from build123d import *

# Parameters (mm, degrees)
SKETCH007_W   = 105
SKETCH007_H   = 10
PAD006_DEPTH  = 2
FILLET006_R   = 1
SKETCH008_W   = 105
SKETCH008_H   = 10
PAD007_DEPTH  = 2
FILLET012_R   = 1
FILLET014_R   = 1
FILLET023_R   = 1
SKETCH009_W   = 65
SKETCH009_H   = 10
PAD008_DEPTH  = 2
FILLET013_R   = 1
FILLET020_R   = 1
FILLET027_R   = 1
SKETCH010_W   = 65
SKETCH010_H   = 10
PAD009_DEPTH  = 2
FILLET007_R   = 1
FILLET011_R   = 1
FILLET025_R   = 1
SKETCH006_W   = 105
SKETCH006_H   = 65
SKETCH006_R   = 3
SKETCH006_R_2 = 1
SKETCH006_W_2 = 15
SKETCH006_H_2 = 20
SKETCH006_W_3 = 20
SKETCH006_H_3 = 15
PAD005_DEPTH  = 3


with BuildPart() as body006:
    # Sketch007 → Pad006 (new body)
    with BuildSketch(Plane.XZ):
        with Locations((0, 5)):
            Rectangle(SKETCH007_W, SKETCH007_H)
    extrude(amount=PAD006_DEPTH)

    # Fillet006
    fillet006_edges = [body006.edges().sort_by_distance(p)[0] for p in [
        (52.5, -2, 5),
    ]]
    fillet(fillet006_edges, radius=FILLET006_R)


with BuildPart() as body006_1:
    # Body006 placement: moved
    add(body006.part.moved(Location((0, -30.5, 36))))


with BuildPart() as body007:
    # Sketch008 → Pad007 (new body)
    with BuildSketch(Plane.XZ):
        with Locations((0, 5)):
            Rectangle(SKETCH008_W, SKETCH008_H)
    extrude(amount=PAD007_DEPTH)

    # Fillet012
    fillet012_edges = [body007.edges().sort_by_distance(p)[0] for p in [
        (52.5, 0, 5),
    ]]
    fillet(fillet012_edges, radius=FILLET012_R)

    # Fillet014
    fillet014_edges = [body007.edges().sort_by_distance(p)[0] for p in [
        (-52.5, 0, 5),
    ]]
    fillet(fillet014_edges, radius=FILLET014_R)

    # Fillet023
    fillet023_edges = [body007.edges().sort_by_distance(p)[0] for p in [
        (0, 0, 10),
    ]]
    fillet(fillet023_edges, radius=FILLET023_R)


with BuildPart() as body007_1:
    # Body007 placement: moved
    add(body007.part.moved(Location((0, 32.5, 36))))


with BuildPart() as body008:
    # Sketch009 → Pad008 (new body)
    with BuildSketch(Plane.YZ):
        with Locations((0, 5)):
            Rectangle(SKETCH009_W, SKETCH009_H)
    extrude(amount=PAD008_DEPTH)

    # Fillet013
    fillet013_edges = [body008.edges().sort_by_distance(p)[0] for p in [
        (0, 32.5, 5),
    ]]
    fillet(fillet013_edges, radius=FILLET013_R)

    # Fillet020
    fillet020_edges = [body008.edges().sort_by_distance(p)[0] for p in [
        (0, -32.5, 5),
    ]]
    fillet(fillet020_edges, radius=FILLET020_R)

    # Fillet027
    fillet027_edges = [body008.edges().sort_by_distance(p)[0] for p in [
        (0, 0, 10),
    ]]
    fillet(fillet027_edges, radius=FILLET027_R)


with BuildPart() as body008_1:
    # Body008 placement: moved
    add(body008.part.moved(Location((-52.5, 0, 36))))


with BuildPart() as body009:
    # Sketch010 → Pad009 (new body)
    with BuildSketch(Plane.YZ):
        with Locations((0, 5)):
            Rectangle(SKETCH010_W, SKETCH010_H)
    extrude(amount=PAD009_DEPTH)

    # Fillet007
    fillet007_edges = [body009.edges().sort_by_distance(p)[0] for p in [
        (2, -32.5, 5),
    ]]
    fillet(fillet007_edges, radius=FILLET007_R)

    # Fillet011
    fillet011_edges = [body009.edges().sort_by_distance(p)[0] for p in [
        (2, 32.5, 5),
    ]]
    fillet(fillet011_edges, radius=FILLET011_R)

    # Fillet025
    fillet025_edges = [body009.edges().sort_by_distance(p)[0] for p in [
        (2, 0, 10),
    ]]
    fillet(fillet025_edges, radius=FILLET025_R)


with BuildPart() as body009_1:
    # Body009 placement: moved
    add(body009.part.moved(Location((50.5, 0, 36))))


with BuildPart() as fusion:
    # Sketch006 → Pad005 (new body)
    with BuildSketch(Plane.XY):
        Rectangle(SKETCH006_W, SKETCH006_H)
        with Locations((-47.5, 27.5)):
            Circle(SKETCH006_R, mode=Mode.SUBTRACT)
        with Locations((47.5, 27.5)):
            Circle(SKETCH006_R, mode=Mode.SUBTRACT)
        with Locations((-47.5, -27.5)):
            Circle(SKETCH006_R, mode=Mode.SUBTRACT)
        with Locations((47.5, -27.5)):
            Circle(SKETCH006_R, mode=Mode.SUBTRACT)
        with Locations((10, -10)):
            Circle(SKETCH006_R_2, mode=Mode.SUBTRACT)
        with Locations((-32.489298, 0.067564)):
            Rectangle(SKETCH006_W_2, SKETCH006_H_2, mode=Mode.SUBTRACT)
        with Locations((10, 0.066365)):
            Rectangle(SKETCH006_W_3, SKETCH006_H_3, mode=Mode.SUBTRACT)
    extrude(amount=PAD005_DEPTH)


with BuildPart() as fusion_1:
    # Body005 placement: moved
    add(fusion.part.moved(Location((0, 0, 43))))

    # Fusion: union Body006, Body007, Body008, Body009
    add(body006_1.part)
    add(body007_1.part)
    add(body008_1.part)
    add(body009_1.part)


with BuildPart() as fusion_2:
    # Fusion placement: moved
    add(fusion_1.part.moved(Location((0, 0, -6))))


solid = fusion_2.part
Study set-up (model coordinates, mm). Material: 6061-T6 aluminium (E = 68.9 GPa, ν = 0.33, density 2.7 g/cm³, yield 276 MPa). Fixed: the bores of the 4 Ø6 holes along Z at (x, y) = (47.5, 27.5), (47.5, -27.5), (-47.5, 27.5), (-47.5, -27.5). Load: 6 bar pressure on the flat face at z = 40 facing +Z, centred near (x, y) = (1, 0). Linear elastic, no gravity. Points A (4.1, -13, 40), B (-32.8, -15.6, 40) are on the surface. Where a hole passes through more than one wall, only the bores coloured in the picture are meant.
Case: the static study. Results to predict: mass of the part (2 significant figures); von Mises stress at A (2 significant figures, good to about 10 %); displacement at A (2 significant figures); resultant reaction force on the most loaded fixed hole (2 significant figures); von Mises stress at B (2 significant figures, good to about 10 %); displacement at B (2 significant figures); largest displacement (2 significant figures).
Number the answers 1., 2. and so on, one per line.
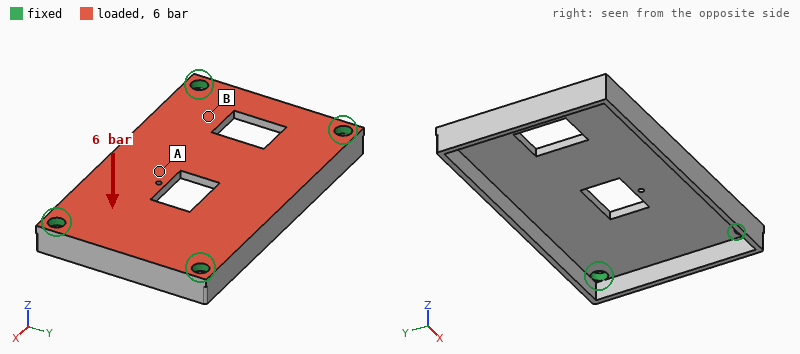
1. 62 g
2. 78 MPa
3. 0.46 mm
4. 960 N
5. 39 MPa
6. 0.18 mm
7. 0.57 mm
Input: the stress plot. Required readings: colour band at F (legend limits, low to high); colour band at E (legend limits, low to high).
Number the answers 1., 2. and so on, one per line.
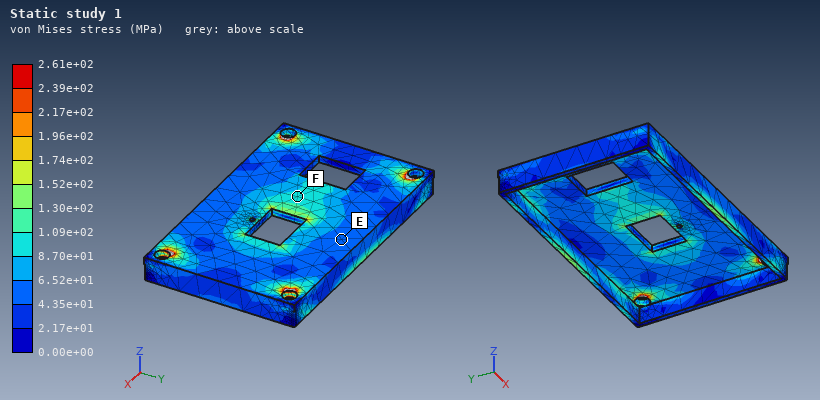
1. 8.70e+01 to 1.09e+02 MPa
2. 4.35e+01 to 6.52e+01 MPa
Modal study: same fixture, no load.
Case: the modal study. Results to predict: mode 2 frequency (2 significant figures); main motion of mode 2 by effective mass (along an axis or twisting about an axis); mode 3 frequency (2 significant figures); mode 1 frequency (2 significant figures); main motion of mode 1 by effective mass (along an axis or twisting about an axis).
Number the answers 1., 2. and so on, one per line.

1. 3900 Hz
2. twisting about X
3. 4900 Hz
4. 2300 Hz
5. along Z
